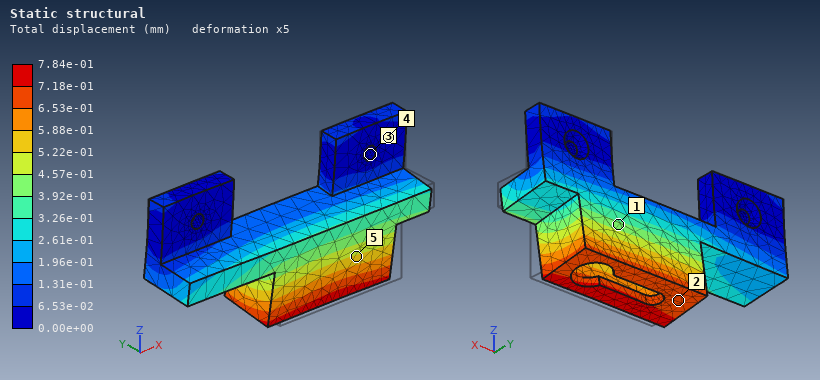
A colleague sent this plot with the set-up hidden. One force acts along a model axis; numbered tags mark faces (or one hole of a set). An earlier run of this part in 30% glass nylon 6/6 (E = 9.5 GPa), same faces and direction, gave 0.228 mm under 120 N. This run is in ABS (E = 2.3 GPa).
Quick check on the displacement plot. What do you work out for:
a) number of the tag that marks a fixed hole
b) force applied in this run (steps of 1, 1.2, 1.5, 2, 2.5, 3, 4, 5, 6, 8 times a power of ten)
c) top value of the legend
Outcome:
3
100 N
7.84e-01 mm
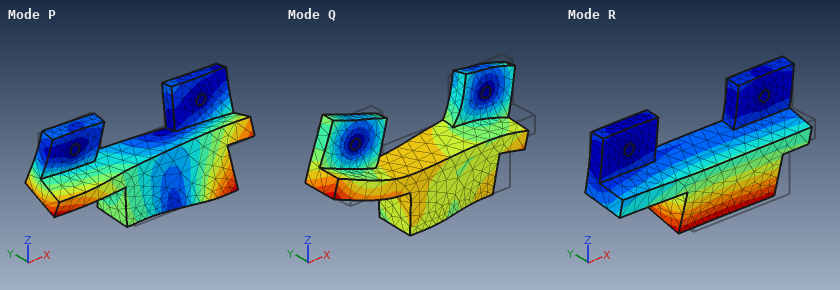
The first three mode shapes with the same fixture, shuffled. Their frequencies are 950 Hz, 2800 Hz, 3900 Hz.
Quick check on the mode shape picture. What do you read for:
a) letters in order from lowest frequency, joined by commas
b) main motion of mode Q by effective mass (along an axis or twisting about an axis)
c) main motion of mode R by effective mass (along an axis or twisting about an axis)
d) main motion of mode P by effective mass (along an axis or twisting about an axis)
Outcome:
R, P, Q
along X
along Y
twisting about Z
